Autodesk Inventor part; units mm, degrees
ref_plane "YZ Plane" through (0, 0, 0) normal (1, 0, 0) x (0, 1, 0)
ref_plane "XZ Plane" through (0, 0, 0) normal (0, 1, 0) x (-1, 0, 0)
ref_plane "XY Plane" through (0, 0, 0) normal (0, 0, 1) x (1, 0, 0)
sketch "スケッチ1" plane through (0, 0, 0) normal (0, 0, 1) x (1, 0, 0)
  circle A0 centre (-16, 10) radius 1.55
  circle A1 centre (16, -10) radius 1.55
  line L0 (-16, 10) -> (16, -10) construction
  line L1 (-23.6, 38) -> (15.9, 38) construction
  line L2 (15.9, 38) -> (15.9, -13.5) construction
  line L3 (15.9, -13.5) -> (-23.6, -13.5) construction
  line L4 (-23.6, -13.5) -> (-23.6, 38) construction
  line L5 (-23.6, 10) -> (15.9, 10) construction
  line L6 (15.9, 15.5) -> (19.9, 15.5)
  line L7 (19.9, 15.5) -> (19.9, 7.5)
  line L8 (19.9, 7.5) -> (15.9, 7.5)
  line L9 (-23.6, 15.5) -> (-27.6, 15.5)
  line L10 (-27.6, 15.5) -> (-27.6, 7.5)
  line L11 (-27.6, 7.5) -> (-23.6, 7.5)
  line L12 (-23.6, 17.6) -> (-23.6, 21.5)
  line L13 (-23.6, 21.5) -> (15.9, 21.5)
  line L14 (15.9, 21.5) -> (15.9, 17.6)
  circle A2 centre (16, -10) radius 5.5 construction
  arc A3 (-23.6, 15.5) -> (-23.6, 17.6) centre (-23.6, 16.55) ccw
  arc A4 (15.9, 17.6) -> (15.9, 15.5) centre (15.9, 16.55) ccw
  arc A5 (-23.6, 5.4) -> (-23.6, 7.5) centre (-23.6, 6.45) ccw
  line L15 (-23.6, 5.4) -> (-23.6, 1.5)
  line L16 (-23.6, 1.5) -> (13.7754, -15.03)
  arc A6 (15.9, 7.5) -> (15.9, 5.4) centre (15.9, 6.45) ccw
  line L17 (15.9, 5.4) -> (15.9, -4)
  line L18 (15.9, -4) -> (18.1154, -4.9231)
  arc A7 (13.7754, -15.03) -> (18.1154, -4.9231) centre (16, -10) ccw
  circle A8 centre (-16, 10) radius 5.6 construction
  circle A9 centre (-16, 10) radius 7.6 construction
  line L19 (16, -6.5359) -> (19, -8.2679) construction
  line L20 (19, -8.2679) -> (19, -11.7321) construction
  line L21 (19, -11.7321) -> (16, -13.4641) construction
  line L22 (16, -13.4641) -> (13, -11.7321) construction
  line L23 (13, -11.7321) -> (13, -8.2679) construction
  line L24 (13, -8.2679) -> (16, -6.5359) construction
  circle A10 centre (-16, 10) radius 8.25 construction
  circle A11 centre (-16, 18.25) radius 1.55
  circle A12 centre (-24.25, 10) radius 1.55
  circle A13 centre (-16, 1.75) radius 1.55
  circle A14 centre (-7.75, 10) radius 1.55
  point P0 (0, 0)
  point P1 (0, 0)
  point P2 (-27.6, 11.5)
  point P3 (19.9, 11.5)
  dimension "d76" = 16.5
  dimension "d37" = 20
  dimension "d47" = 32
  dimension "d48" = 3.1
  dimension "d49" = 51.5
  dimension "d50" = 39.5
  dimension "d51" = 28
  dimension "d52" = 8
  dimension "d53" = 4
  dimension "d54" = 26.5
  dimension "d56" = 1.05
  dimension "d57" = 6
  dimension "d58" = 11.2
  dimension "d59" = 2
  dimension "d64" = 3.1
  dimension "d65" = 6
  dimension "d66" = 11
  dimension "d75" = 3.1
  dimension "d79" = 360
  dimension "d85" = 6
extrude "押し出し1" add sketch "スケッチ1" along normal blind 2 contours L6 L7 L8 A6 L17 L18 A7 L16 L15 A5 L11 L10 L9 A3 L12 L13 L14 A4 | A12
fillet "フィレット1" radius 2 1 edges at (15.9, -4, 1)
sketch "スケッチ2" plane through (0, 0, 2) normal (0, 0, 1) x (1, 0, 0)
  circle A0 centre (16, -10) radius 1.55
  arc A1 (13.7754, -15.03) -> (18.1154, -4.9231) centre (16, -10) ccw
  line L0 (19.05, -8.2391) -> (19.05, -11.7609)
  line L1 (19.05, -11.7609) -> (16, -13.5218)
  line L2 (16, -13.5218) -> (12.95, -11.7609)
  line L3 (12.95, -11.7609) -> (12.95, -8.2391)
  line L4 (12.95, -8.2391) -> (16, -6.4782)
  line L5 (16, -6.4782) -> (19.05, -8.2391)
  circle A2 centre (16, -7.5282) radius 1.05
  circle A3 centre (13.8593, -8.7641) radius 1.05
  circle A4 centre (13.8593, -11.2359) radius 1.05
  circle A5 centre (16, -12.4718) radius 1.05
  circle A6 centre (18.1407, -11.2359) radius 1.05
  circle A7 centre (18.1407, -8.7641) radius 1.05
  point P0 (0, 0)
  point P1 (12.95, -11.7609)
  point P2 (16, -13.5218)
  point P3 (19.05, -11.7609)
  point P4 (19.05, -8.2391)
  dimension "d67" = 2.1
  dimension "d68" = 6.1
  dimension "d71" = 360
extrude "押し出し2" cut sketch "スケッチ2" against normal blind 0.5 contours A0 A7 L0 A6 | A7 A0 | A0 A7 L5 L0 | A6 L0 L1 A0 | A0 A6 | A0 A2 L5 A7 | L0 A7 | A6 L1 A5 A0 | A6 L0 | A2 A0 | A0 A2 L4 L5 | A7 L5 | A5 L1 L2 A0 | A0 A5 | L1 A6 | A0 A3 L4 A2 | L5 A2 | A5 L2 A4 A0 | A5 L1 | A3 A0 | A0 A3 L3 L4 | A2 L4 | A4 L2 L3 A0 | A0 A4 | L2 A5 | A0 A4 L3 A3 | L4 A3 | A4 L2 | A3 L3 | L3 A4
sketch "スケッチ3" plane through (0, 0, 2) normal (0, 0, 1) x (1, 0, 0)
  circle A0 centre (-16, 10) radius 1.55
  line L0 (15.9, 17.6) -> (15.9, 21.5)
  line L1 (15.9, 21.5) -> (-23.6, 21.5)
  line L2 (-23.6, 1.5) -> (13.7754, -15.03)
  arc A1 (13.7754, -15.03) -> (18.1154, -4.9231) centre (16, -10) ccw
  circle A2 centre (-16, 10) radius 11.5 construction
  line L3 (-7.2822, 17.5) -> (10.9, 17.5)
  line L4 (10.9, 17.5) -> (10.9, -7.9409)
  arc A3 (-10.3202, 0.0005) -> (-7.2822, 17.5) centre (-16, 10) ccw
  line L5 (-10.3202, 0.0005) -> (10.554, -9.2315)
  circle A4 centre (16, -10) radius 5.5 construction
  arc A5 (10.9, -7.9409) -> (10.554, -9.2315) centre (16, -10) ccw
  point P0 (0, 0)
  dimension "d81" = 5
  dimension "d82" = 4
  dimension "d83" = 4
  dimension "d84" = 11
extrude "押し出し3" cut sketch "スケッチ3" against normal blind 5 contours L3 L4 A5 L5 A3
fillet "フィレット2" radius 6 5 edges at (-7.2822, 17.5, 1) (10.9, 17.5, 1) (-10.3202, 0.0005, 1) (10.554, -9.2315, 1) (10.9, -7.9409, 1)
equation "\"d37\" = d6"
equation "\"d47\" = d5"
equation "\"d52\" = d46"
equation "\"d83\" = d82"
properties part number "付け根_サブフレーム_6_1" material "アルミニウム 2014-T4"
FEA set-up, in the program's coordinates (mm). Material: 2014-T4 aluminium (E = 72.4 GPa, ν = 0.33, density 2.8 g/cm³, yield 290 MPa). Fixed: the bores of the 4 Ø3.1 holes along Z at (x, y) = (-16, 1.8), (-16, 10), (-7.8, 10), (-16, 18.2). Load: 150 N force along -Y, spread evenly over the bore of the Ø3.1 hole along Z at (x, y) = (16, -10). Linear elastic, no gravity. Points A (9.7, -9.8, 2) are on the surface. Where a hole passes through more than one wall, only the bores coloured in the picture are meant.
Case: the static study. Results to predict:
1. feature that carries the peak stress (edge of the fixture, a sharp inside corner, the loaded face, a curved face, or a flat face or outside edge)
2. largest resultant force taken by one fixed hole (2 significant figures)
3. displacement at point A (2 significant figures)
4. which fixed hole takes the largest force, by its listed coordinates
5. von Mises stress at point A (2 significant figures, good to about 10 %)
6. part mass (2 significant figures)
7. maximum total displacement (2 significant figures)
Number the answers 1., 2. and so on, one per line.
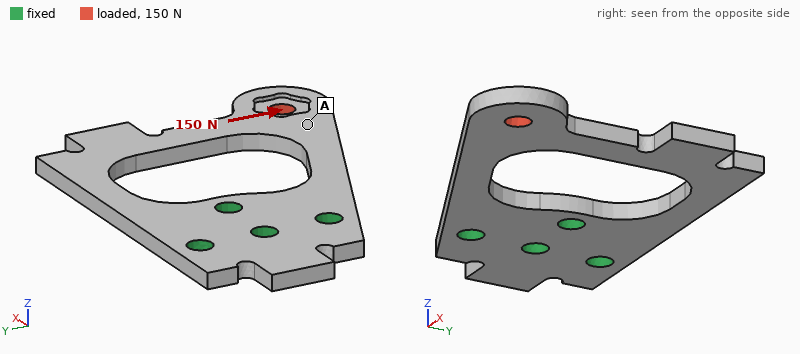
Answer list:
1. a curved face
2. 280 N
3. 66 µm
4. (-7.8, 10)
5. 13 MPa
6. 4.8 g
7. 98 µm
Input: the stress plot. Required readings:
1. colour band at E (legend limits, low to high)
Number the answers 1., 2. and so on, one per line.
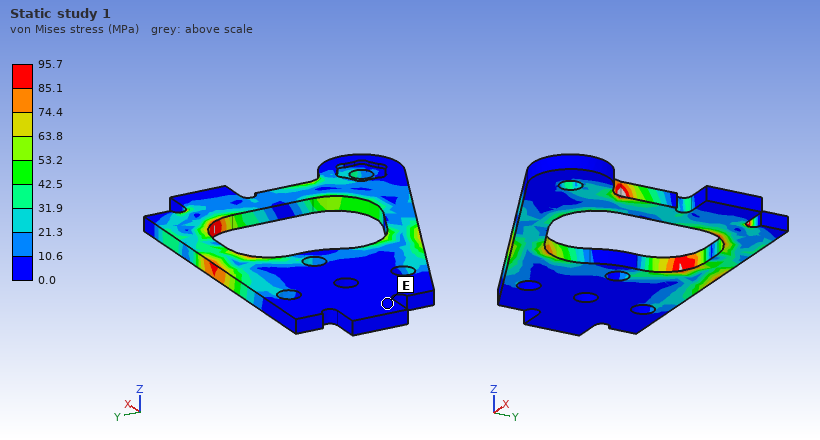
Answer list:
1. 0.0 to 10.6 MPa
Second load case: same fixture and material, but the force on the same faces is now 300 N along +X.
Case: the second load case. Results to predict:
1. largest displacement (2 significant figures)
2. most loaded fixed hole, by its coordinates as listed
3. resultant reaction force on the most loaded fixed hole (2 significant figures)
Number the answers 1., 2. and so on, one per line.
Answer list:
1. 0.13 mm
2. (-16, 1.8)
3. 410 N
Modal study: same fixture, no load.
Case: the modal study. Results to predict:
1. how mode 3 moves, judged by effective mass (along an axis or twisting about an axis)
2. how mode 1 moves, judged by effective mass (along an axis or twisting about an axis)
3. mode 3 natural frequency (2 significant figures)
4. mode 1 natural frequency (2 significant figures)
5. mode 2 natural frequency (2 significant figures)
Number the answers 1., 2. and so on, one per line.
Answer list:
1. along Y
2. along Z
3. 5600 Hz
4. 1100 Hz
5. 2400 Hz
